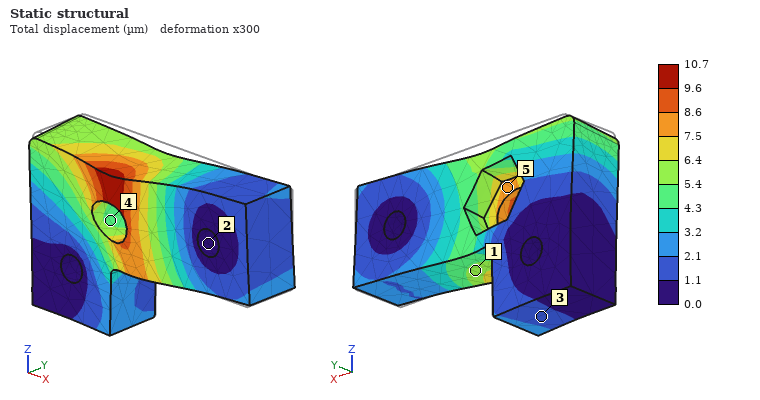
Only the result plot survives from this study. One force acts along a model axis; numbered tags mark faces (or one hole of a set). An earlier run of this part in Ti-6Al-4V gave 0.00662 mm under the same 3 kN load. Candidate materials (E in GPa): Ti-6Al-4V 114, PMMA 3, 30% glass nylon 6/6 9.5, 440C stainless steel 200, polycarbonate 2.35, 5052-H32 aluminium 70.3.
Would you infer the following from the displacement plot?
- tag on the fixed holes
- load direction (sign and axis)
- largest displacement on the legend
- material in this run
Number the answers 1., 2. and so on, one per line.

1. 2
2. -Z
3. 10.7 µm
4. 5052-H32 aluminium
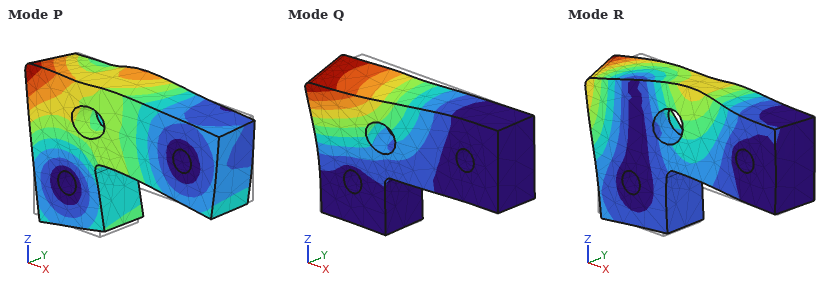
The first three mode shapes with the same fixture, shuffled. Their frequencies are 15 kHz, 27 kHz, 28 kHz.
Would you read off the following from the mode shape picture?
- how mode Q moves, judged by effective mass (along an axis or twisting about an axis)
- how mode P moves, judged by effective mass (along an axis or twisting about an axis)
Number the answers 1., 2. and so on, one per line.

1. along Y
2. along X
